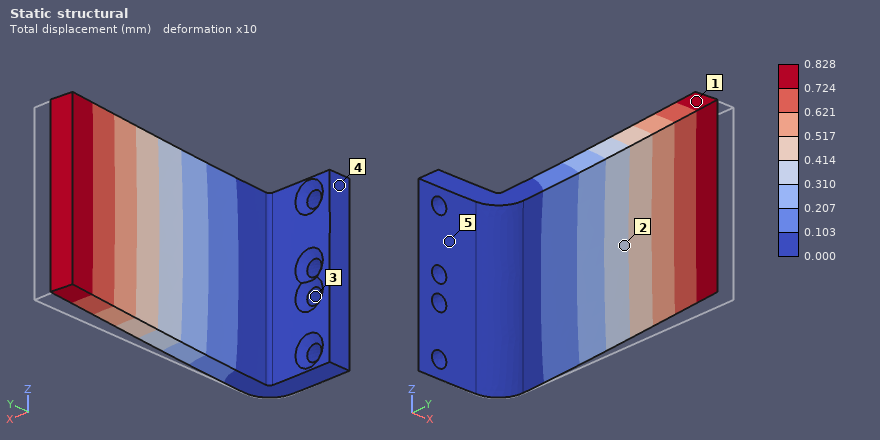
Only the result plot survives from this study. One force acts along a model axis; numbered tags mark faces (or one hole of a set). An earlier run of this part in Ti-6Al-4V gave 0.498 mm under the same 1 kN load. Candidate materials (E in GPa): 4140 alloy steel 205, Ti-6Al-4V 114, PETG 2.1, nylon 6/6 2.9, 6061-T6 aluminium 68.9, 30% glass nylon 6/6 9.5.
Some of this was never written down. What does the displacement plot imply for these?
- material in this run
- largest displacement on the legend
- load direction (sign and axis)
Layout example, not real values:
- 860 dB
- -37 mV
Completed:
- 6061-T6 aluminium
- 0.828 mm
- -X
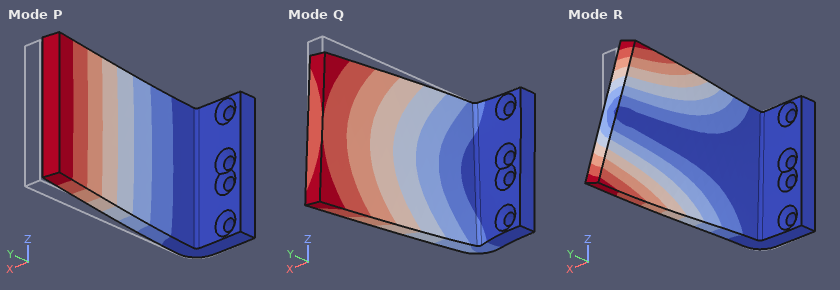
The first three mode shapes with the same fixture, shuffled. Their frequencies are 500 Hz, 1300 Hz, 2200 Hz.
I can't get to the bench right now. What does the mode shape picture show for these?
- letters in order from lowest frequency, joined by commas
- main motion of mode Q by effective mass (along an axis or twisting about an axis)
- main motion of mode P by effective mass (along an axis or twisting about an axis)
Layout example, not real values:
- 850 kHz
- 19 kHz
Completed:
- P, Q, R
- along Z
- along X
